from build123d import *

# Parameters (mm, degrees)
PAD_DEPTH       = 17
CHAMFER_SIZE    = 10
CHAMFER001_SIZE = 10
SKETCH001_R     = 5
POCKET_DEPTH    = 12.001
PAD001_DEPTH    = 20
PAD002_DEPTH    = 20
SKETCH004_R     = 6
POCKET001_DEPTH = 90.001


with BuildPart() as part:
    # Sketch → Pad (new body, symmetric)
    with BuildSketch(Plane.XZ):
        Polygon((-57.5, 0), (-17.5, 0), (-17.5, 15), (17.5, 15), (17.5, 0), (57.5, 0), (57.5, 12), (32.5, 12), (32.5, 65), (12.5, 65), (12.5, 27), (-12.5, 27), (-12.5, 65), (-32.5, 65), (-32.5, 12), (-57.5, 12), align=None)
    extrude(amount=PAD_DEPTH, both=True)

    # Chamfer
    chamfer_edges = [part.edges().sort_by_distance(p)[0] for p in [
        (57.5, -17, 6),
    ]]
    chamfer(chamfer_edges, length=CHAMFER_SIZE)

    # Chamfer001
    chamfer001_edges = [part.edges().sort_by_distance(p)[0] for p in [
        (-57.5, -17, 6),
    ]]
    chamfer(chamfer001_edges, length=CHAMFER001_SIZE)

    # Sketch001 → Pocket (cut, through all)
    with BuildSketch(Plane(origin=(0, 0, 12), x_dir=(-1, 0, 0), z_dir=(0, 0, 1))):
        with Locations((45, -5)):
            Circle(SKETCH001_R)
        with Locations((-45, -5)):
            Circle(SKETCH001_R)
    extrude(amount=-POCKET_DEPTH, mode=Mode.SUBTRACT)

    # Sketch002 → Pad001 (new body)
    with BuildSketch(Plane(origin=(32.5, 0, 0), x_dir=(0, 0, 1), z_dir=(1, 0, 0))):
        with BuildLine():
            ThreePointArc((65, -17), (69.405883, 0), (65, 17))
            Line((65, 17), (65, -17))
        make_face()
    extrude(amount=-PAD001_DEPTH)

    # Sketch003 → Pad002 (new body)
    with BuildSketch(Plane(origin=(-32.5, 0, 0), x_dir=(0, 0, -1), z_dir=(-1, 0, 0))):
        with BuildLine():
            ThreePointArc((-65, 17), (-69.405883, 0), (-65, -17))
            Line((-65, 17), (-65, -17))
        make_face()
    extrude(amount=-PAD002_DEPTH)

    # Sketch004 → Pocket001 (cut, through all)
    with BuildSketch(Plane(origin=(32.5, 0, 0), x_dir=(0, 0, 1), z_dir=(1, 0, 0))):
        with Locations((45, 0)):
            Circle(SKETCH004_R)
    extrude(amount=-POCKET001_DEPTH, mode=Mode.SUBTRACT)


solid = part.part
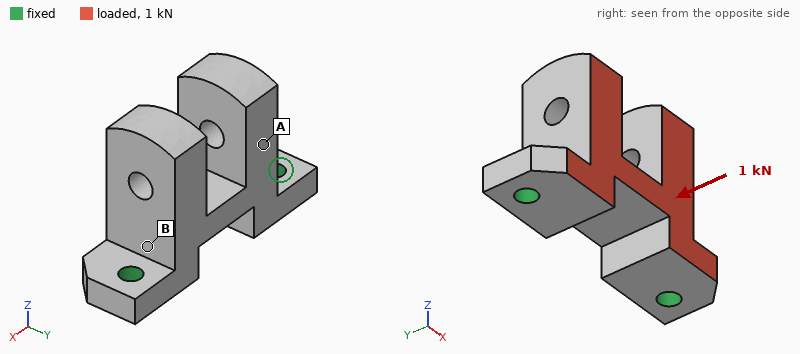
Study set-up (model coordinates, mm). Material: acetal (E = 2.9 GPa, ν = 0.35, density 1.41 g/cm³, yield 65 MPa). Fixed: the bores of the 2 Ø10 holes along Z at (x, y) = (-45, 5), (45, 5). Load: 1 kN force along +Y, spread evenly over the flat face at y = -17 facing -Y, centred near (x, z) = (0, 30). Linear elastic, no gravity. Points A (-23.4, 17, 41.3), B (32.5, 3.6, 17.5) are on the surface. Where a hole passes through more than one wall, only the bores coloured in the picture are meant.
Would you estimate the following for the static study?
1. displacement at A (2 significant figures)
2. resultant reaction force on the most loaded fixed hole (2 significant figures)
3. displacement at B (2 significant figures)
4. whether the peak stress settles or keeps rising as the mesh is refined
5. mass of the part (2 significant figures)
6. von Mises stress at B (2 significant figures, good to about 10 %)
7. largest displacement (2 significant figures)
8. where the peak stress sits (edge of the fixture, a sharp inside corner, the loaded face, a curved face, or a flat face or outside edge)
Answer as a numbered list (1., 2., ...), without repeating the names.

1. 0.43 mm
2. 500 N
3. 0.15 mm
4. keeps rising
5. 160 g
6. 4.8 MPa
7. 0.71 mm
8. edge of the fixture
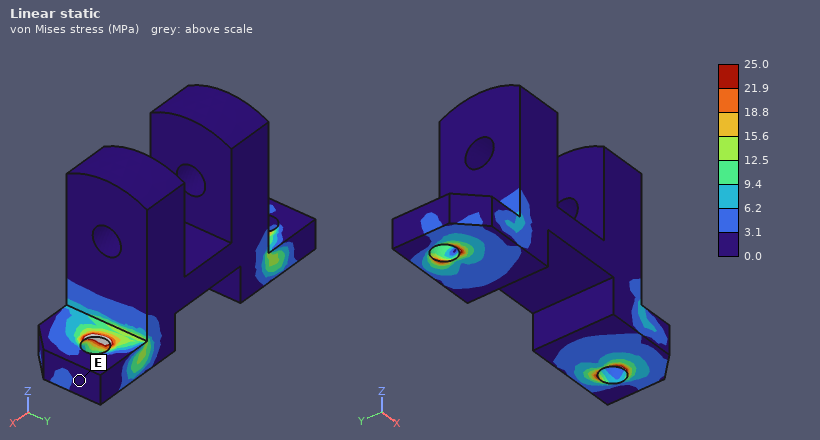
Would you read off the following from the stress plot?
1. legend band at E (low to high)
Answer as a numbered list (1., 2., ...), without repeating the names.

1. 0.0 to 3.1 MPa
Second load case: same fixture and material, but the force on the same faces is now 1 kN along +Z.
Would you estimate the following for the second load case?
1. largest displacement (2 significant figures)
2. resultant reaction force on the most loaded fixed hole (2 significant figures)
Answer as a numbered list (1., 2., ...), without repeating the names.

1. 0.56 mm
2. 610 N
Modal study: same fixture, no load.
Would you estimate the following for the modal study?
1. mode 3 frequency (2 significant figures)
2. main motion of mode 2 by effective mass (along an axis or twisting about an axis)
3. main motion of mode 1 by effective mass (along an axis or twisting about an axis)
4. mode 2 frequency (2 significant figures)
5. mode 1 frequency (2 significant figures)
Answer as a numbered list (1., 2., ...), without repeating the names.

1. 1200 Hz
2. twisting about Z
3. along Y
4. 980 Hz
5. 580 Hz
